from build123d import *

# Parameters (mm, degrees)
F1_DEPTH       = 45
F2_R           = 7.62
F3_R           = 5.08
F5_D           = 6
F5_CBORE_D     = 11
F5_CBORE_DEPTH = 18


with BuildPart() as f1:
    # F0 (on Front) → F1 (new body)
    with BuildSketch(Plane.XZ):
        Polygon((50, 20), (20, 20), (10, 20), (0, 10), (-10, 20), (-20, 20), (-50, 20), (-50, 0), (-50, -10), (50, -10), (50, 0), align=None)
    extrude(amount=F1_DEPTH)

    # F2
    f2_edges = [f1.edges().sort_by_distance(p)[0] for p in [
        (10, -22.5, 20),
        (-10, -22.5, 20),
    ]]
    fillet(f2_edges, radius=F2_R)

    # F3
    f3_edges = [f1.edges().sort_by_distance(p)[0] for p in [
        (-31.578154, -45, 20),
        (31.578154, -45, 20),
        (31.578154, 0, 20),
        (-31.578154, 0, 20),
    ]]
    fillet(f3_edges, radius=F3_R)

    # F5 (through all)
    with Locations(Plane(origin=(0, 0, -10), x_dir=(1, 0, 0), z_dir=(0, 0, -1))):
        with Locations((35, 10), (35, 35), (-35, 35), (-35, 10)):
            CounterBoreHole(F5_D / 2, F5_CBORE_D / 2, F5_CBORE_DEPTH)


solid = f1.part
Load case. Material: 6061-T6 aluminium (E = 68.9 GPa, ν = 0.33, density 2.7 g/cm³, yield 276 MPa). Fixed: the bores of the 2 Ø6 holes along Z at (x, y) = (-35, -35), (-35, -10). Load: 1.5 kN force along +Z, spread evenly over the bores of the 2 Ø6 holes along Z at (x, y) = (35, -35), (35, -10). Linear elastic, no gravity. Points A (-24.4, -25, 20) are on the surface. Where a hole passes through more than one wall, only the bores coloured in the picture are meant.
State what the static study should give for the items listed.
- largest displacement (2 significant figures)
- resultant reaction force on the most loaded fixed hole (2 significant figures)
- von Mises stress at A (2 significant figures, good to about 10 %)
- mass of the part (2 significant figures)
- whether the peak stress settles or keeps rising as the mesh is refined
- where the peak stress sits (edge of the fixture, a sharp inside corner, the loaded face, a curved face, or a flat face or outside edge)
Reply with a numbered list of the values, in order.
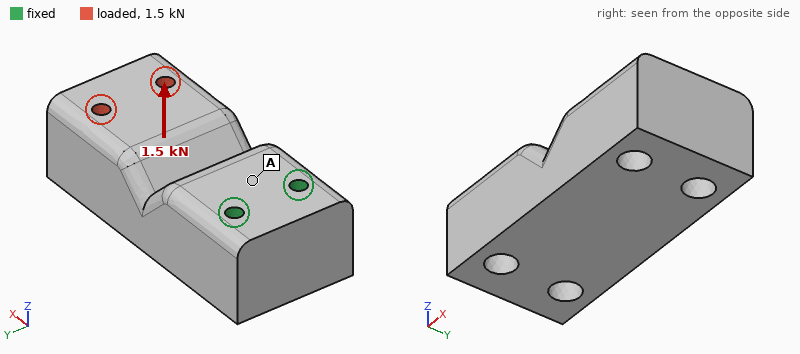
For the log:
1. 0.14 mm
2. 810 N
3. 16 MPa
4. 330 g
5. keeps rising
6. edge of the fixture
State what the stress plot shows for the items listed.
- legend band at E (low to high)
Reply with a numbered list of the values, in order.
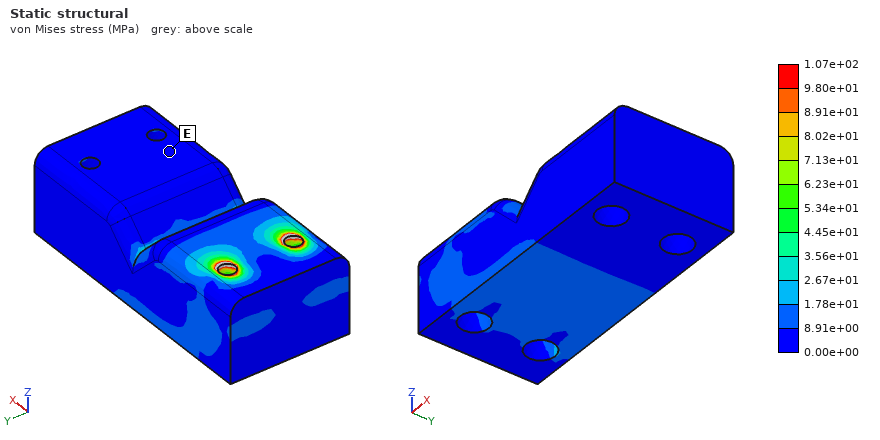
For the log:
1. 0.00e+00 to 8.91e+00 MPa
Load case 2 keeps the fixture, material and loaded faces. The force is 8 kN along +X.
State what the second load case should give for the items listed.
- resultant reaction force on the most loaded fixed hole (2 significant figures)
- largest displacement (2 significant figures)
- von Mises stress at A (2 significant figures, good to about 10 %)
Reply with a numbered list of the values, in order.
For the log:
1. 4.0 kN
2. 74 µm
3. 12 MPa
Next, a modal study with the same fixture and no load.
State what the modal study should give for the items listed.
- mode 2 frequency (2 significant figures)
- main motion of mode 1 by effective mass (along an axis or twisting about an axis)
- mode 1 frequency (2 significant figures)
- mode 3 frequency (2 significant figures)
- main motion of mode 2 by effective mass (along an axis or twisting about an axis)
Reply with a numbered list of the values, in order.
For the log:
1. 3100 Hz
2. along Z
3. 1600 Hz
4. 6600 Hz
5. along Y
